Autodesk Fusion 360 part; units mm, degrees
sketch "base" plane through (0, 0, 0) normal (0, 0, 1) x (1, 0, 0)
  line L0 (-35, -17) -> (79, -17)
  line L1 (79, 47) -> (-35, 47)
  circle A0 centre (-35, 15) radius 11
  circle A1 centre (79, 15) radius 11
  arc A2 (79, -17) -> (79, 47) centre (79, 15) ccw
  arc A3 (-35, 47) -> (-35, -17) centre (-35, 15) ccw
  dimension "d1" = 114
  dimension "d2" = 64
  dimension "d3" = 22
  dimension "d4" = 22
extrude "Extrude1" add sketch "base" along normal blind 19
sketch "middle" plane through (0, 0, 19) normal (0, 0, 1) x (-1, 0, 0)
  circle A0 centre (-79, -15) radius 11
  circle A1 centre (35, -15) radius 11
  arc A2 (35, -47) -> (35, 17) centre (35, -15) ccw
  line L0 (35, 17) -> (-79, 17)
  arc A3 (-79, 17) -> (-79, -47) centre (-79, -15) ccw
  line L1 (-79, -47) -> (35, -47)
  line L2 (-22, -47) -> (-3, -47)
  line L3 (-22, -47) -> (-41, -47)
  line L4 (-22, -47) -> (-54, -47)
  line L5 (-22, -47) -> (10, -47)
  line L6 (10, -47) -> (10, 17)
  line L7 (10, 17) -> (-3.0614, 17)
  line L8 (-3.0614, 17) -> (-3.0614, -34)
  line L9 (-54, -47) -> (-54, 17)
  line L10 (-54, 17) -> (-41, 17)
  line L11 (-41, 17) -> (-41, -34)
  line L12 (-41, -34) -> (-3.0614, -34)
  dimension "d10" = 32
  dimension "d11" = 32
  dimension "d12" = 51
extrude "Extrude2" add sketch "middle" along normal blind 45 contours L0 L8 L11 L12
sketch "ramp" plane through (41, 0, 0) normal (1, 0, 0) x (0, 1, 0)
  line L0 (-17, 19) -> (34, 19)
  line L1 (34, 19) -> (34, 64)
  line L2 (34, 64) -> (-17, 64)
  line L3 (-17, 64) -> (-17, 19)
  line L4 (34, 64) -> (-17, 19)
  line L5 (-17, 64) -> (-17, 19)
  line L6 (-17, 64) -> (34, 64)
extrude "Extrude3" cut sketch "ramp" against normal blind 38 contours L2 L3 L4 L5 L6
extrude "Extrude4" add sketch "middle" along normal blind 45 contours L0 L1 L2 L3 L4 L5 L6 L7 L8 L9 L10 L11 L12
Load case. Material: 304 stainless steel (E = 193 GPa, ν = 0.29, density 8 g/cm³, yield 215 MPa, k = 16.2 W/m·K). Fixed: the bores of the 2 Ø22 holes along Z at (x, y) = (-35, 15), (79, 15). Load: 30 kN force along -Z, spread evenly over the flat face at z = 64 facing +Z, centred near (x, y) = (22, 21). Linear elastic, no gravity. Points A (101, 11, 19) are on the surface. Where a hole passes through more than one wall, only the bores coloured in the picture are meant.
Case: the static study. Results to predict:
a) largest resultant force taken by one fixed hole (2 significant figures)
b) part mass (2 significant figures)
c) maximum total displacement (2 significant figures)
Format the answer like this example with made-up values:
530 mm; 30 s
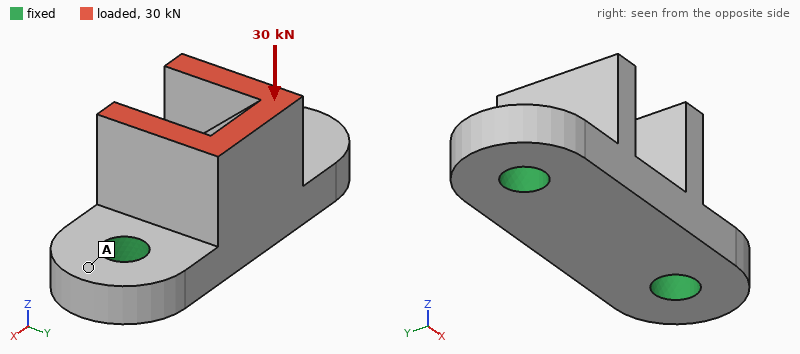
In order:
16 kN; 2.6 kg; 23 µm
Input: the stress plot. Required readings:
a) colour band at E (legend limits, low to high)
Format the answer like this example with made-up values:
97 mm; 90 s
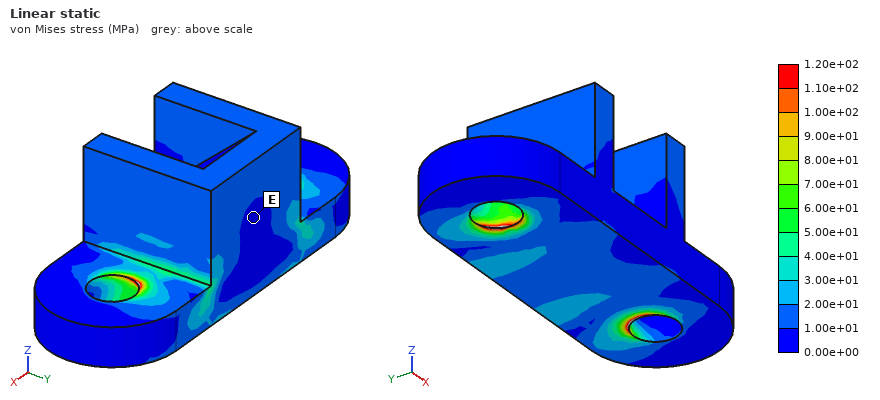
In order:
0.00e+00 to 1.00e+01 MPa
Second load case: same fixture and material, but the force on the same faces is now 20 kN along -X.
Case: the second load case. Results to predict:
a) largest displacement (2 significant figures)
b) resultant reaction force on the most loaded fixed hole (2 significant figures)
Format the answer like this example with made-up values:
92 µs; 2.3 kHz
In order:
52 µm; 16 kN
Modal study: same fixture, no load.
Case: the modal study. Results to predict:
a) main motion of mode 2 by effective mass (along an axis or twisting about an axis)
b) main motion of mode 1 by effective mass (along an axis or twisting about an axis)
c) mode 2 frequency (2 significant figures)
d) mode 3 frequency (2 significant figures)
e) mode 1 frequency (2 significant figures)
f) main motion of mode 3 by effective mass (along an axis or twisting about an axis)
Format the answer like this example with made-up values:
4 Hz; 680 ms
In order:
along Z; along Y; 6100 Hz; 6900 Hz; 3400 Hz; along X
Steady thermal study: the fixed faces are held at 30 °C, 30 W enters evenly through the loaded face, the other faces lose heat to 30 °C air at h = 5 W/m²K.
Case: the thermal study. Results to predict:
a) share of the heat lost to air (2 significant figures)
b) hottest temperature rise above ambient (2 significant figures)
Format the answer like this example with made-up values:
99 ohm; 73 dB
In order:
12 %; 53 K
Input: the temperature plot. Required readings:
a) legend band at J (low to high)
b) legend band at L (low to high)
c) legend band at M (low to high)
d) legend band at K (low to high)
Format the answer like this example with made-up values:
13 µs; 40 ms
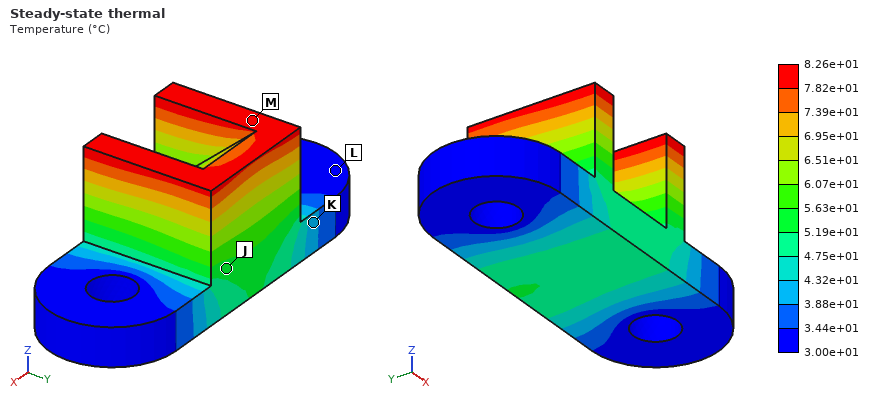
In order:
5.19e+01 to 5.63e+01 °C; 3.00e+01 to 3.44e+01 °C; 7.82e+01 to 8.26e+01 °C; 3.88e+01 to 4.32e+01 °C
